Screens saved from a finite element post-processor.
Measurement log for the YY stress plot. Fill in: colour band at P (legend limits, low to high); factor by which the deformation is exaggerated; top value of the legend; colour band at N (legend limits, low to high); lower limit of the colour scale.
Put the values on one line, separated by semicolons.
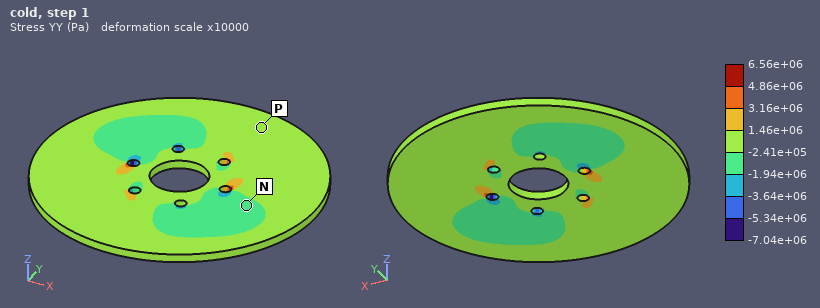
-2.41e+05 to 1.46e+06 Pa; 10000; 6.56e+06 Pa; -1.94e+06 to -2.41e+05 Pa; -7.04e+06 Pa
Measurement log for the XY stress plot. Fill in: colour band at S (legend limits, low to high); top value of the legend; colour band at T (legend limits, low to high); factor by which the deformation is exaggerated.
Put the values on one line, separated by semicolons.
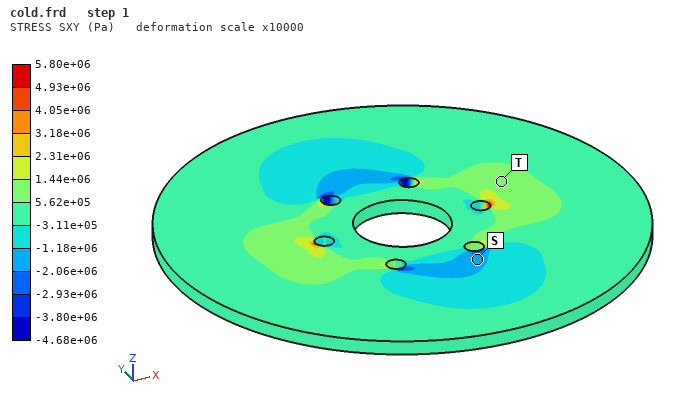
-2.06e+06 to -1.18e+06 Pa; 5.80e+06 Pa; 5.62e+05 to 1.44e+06 Pa; 10000
